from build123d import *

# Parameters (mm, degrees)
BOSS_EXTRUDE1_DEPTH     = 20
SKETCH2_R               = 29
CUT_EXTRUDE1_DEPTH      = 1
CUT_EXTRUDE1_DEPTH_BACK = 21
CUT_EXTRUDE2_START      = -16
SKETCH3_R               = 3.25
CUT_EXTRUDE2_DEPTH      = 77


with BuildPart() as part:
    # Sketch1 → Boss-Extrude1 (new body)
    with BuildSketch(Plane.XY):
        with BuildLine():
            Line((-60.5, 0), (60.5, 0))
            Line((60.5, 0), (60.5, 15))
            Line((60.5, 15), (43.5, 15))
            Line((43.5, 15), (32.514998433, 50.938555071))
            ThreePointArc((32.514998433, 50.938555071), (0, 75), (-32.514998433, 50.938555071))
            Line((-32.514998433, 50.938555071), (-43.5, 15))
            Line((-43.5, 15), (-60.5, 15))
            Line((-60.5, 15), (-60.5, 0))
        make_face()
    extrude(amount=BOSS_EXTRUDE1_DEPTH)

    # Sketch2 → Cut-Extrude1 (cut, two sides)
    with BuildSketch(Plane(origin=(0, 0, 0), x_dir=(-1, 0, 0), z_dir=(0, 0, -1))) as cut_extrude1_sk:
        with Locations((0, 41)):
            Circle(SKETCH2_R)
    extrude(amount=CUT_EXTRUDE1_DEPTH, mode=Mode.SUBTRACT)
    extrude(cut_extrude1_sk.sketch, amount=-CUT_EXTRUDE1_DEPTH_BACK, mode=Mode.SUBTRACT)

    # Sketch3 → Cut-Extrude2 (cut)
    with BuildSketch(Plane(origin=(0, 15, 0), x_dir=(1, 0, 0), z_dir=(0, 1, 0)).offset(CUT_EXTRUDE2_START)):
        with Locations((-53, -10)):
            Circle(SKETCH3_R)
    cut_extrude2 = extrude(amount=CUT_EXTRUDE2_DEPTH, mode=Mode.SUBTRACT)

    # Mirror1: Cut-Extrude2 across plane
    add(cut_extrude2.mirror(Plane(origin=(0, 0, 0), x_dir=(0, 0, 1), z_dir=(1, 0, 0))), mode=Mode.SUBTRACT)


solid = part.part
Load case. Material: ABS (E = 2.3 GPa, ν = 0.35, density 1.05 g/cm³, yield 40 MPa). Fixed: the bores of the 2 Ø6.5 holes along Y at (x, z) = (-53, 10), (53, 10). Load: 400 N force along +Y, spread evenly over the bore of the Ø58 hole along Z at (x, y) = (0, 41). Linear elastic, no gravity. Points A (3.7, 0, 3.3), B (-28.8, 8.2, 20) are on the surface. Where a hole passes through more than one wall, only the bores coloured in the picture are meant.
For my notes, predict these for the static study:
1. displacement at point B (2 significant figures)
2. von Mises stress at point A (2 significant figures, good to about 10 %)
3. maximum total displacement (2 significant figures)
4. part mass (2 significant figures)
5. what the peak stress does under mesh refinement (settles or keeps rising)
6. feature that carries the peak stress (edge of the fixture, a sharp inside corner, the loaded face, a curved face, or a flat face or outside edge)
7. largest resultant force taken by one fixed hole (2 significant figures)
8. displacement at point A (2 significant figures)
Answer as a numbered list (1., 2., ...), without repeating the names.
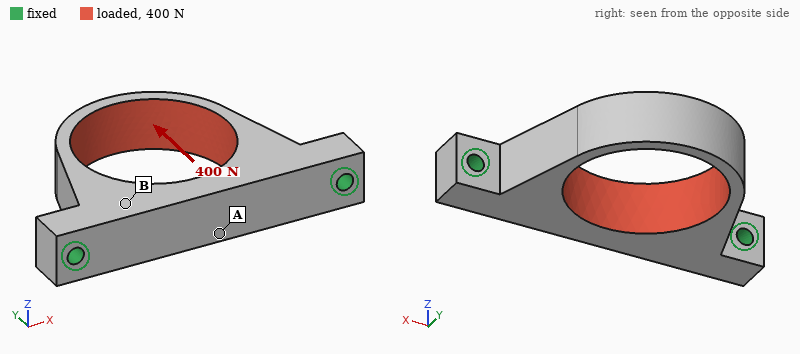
1. 44 µm
2. 1.6 MPa
3. 82 µm
4. 63 g
5. keeps rising
6. edge of the fixture
7. 200 N
8. 79 µm
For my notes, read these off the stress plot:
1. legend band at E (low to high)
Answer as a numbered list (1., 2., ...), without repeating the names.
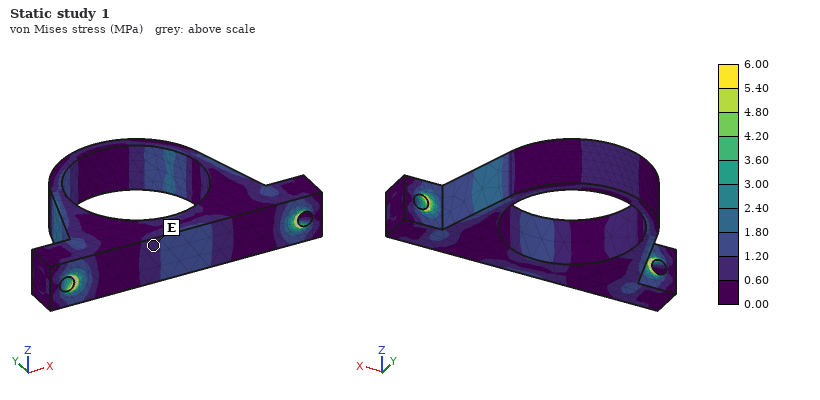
1. 0.60 to 1.20 MPa
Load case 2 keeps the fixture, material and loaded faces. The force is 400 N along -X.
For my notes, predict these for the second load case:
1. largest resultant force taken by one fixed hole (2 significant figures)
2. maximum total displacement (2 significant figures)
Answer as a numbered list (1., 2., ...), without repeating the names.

1. 240 N
2. 0.46 mm
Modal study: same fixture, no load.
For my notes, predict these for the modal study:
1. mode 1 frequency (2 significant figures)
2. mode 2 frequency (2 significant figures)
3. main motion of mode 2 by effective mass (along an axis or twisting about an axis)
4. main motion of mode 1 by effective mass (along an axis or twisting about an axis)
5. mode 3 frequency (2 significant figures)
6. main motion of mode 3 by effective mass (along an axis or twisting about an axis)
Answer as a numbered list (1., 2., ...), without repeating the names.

1. 750 Hz
2. 1100 Hz
3. along X
4. along Z
5. 1500 Hz
6. along Y
